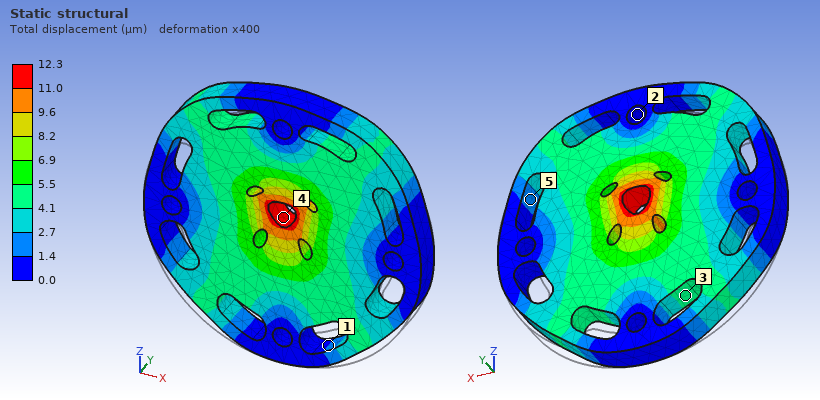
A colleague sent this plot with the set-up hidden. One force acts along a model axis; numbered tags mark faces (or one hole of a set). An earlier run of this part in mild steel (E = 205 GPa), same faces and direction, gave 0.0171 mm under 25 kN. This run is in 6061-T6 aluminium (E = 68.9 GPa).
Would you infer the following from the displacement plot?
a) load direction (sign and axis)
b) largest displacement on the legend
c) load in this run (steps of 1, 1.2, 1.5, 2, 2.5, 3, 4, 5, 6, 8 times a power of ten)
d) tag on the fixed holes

+Z
12.3 µm
6 kN
2
